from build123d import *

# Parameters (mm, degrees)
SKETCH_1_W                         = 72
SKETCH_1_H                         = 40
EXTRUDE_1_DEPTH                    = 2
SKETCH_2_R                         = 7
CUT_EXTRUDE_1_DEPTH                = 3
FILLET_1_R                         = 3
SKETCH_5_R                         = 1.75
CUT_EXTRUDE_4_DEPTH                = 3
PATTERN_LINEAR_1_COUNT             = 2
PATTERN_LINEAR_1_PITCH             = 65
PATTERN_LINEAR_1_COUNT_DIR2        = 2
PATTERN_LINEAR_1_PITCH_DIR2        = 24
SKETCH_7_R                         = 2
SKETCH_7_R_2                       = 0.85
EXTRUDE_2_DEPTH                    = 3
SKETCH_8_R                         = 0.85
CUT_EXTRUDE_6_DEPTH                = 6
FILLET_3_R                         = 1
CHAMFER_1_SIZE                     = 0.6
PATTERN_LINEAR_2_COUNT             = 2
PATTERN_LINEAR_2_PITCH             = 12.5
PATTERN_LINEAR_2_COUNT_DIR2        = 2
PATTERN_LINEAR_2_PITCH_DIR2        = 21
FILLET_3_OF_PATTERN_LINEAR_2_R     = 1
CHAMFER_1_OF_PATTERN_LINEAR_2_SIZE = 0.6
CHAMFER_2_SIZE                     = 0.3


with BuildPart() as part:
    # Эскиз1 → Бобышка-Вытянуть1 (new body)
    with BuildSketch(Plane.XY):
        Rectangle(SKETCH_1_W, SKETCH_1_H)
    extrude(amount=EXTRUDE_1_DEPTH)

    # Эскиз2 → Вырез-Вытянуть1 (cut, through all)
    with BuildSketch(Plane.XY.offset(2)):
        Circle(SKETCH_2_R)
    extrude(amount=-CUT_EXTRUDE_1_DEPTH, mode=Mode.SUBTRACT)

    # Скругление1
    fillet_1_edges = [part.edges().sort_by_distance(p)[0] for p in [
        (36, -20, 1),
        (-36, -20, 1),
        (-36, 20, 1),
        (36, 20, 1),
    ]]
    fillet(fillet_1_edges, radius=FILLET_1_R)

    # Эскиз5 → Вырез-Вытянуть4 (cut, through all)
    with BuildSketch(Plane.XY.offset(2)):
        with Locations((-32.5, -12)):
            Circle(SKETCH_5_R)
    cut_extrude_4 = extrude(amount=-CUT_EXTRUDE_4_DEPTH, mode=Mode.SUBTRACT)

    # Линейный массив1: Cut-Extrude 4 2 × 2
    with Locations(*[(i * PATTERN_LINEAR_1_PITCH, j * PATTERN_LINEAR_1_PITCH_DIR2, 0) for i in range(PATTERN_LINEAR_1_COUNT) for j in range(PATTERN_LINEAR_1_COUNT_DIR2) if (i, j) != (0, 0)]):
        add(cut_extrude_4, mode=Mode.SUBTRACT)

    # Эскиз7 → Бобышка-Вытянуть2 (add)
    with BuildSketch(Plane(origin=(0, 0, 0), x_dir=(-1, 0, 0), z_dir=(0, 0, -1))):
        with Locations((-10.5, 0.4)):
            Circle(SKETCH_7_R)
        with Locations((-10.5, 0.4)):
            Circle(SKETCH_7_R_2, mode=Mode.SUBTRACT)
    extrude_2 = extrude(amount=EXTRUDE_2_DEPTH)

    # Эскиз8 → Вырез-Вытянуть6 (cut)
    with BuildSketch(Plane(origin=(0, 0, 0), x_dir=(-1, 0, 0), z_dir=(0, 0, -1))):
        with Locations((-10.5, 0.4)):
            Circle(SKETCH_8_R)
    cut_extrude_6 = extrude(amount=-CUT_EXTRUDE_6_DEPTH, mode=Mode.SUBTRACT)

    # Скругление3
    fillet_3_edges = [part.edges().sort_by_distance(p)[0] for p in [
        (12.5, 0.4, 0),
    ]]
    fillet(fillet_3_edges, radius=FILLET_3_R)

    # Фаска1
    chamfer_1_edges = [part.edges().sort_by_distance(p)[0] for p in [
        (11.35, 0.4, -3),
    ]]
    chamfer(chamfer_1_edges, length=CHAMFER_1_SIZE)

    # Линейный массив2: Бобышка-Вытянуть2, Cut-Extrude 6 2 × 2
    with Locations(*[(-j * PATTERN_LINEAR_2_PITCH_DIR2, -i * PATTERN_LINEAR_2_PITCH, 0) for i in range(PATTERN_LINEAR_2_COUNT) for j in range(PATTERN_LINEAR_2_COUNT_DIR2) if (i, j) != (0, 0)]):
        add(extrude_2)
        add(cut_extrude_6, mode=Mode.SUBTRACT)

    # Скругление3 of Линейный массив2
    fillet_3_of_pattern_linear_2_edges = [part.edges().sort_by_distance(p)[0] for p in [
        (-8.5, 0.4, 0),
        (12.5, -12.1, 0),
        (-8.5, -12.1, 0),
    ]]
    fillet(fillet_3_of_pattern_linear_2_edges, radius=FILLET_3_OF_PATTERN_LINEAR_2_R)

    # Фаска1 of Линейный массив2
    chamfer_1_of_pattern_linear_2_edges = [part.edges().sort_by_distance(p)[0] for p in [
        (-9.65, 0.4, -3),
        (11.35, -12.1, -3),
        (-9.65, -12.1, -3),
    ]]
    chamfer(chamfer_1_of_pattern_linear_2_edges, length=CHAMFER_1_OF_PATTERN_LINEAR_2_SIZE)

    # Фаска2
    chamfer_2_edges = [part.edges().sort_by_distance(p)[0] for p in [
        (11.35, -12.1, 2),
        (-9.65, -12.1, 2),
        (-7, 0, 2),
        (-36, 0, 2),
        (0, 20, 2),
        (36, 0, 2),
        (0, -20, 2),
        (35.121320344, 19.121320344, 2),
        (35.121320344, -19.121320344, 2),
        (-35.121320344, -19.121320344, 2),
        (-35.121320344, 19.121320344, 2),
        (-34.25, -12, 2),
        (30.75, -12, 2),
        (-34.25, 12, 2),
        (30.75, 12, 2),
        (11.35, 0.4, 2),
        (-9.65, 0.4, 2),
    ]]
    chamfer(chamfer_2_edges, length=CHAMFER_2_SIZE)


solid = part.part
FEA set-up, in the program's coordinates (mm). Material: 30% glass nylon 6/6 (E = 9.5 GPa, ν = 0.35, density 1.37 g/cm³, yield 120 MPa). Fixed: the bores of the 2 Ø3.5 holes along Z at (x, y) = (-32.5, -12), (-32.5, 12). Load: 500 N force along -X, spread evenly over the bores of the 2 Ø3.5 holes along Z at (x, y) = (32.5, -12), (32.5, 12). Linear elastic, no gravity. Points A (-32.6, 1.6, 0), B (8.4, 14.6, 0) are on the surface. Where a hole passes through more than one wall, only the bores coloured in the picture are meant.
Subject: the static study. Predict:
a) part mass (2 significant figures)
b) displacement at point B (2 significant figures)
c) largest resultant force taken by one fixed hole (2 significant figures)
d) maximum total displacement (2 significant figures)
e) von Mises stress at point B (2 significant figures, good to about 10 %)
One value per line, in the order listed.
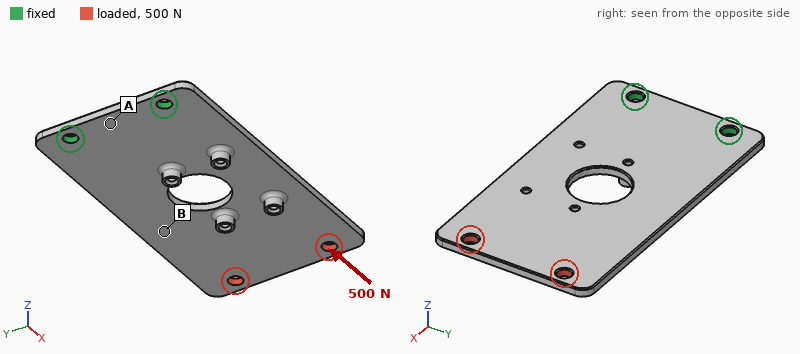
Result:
7.5 g
0.25 mm
250 N
0.73 mm
12 MPa
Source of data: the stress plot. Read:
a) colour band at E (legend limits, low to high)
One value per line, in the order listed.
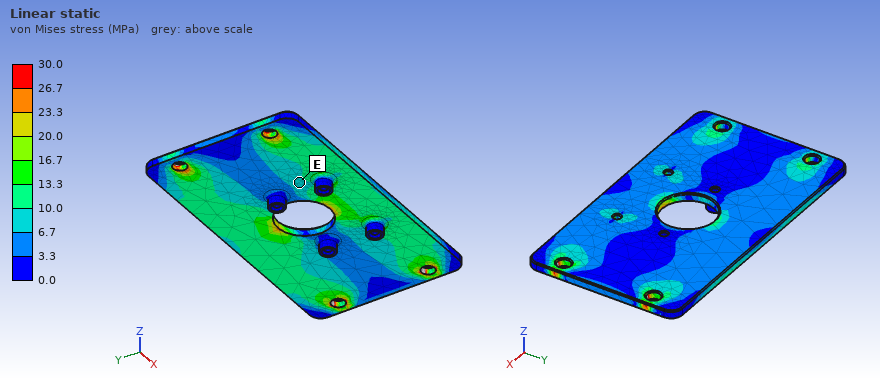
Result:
6.7 to 10.0 MPa
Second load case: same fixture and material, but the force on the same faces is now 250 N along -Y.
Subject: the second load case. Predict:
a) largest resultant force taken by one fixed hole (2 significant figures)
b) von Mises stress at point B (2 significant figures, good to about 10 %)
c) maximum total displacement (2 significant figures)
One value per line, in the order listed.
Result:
630 N
8.6 MPa
0.47 mm
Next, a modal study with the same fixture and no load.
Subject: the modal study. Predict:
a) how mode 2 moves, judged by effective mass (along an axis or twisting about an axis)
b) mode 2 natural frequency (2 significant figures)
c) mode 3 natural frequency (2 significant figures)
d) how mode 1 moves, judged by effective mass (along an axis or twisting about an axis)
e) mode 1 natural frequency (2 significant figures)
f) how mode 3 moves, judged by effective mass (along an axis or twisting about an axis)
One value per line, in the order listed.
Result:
twisting about X
660 Hz
1100 Hz
along Z
180 Hz
along Z
